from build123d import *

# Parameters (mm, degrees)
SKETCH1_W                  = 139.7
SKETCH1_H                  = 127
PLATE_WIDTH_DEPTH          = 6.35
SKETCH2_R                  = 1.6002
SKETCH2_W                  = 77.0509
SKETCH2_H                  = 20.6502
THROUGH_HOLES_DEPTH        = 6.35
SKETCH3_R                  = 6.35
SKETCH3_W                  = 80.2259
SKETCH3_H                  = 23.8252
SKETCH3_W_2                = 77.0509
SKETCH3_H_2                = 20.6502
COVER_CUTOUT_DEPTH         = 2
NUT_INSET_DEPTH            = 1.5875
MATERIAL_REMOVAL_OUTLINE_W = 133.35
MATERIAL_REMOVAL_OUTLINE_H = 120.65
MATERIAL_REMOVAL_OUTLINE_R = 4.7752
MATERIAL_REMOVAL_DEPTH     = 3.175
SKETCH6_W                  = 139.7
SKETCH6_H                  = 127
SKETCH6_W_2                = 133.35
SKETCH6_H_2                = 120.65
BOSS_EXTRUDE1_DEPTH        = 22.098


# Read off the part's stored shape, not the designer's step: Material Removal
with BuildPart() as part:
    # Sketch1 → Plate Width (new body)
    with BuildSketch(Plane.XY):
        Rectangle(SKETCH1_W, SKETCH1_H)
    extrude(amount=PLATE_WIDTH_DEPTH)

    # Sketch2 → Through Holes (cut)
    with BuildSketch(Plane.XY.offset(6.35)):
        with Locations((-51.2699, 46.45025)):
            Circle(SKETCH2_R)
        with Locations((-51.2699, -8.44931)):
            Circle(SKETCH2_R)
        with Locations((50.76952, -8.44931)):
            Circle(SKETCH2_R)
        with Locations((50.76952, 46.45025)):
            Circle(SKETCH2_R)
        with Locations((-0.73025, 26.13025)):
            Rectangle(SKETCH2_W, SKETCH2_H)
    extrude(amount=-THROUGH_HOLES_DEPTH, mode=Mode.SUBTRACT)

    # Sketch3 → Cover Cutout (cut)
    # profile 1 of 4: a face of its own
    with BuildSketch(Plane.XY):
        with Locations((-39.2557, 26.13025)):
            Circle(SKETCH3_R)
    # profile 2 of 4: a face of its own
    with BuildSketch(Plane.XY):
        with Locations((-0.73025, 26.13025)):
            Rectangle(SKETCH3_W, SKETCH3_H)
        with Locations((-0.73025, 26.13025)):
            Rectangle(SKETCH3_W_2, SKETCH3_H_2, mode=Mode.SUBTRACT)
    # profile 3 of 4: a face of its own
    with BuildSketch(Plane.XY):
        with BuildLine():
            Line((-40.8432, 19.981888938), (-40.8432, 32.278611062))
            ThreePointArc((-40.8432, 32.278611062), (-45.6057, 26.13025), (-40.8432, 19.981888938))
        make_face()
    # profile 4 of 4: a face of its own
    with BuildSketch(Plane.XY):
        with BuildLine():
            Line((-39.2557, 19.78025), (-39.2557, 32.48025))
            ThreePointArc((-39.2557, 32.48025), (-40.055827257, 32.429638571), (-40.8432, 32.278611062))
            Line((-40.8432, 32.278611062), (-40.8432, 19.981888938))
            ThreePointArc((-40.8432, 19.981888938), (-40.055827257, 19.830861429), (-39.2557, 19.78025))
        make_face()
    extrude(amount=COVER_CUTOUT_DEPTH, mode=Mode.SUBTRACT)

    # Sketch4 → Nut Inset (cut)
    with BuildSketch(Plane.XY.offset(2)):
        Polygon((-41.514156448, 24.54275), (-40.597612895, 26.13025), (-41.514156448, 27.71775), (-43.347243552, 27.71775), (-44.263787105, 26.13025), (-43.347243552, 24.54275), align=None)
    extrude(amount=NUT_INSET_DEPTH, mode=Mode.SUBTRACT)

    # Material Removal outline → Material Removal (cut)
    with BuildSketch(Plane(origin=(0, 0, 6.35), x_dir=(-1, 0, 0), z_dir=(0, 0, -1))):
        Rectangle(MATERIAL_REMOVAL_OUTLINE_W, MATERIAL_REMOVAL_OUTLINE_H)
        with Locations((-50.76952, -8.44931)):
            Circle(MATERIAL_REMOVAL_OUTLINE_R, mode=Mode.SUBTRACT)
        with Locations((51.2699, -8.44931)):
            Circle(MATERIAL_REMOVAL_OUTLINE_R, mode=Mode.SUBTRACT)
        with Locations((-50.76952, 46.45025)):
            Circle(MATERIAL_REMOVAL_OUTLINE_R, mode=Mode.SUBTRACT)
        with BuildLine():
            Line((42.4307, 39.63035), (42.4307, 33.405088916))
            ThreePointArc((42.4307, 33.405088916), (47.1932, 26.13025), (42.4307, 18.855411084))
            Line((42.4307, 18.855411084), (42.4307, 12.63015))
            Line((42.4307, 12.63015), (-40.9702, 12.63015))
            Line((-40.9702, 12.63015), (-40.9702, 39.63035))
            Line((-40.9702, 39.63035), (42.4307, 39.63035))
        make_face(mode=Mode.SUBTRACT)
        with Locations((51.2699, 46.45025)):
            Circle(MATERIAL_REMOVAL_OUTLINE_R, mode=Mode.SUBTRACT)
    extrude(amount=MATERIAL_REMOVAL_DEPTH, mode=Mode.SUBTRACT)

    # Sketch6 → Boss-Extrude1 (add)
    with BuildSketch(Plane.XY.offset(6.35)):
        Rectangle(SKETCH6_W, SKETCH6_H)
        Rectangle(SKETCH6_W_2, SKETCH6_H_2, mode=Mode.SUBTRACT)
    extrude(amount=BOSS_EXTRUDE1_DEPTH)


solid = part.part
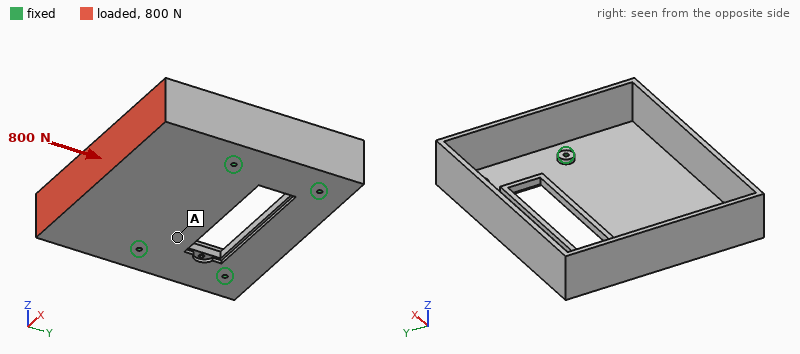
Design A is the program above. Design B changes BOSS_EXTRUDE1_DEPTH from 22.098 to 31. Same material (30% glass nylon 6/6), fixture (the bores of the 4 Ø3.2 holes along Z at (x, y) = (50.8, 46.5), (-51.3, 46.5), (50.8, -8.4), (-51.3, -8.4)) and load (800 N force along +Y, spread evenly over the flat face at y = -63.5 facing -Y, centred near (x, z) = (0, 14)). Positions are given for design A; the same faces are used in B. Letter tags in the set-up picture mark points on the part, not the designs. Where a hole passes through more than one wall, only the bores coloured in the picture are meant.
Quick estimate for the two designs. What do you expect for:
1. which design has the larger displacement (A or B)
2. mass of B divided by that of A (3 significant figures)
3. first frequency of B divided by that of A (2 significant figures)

B
1.15
0.94
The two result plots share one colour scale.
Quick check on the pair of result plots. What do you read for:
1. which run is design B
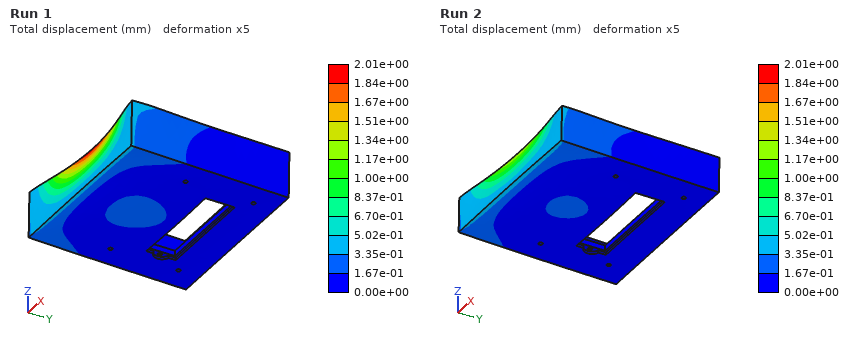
Run 1
